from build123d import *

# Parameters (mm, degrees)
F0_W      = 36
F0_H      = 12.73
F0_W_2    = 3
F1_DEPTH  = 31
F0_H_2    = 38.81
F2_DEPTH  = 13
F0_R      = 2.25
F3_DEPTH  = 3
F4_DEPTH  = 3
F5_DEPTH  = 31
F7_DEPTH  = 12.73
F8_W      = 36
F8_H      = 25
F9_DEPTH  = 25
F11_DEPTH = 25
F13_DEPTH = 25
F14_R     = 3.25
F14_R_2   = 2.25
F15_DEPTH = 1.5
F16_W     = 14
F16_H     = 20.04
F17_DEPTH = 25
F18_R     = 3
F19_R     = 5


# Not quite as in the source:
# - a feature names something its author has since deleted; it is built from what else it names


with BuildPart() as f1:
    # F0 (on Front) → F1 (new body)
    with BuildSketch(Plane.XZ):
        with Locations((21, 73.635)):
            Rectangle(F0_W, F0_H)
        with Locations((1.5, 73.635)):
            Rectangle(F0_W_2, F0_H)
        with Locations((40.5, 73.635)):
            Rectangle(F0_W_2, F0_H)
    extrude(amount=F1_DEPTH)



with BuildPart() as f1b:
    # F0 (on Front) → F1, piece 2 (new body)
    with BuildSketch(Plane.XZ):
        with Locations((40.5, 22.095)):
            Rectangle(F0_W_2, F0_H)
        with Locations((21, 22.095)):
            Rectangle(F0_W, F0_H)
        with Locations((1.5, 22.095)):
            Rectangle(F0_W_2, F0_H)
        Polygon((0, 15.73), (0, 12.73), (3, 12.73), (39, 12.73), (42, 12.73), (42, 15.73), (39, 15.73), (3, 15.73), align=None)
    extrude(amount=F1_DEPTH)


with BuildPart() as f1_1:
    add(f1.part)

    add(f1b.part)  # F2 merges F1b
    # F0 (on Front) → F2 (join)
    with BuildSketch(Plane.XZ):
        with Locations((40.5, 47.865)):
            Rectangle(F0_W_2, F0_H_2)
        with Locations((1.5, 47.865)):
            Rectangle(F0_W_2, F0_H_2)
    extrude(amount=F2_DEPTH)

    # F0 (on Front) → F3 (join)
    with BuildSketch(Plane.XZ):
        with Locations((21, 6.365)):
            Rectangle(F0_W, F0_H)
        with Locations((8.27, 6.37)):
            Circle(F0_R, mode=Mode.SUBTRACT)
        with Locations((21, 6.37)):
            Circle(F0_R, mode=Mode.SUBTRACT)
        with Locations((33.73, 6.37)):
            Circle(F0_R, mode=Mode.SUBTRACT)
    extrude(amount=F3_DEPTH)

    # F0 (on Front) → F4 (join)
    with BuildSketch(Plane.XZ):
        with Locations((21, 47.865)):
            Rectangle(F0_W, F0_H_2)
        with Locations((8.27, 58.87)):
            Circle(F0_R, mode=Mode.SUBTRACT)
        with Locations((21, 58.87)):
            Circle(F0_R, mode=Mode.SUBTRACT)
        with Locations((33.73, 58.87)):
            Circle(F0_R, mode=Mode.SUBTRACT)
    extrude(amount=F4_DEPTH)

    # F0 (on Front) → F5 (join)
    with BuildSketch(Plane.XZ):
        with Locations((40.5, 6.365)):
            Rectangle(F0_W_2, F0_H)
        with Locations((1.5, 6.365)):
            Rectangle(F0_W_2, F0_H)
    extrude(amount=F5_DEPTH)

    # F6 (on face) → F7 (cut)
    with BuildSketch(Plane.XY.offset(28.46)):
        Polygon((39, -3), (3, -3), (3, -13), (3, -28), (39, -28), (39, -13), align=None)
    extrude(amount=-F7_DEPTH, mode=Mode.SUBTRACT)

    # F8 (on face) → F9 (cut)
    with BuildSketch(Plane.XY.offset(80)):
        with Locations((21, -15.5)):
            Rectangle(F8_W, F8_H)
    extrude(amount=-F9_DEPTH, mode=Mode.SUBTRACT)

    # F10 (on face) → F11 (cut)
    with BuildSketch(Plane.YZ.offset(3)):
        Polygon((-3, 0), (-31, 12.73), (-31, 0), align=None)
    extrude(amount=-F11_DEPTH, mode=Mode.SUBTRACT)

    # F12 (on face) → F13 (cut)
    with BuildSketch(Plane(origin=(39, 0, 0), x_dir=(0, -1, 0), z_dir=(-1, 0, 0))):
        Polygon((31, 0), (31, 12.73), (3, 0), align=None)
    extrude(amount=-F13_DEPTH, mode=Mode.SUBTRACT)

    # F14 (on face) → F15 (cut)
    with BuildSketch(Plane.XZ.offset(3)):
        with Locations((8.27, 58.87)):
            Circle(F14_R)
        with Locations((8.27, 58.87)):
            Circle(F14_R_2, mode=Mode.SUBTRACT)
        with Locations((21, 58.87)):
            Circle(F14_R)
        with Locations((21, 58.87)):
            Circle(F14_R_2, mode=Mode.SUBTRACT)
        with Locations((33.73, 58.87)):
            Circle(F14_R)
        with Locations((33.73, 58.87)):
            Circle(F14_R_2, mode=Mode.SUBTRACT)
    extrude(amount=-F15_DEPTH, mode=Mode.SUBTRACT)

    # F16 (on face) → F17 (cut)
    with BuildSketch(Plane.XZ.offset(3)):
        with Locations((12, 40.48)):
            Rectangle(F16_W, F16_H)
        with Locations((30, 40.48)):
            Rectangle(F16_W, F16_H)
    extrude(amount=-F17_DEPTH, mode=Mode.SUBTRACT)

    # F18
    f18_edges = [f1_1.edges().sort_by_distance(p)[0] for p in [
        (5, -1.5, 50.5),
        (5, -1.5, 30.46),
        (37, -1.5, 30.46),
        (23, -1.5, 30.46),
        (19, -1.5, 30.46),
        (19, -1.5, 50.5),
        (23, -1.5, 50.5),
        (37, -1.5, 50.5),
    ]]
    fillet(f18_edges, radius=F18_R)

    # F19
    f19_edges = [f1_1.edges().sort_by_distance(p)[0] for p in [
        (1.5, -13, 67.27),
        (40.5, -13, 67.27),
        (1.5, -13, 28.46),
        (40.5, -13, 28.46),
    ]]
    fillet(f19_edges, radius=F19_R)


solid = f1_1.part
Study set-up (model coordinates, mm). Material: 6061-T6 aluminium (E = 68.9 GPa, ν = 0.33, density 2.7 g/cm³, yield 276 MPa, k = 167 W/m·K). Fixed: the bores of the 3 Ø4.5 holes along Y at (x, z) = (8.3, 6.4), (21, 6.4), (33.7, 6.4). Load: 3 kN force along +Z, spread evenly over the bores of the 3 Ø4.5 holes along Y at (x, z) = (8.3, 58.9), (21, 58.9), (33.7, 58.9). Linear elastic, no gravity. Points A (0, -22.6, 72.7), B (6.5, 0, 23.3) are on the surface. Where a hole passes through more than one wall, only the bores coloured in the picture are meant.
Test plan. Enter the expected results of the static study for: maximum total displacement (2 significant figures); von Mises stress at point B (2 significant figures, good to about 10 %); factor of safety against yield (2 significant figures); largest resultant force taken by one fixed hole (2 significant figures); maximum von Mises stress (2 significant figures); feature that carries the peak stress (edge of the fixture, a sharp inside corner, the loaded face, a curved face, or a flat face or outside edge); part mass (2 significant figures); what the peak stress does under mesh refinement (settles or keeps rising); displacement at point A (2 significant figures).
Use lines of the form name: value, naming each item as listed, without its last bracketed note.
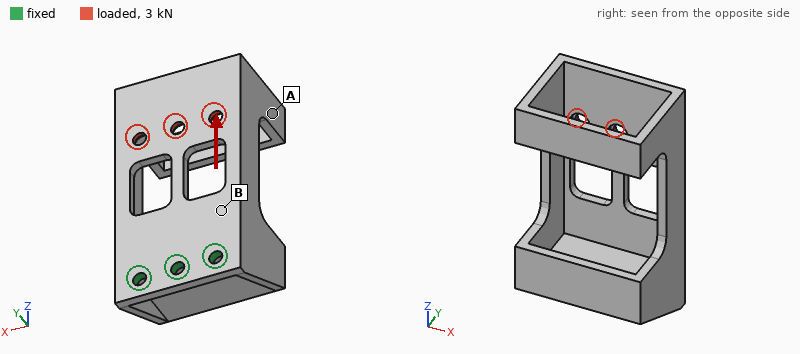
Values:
maximum total displacement: 0.25 mm
von Mises stress at point B: 29 MPa
factor of safety against yield: 1.9
largest resultant force taken by one fixed hole: 1.2 kN
maximum von Mises stress: 150 MPa
feature that carries the peak stress: a curved face
part mass: 60 g
what the peak stress does under mesh refinement: settles
displacement at point A: 0.20 mm
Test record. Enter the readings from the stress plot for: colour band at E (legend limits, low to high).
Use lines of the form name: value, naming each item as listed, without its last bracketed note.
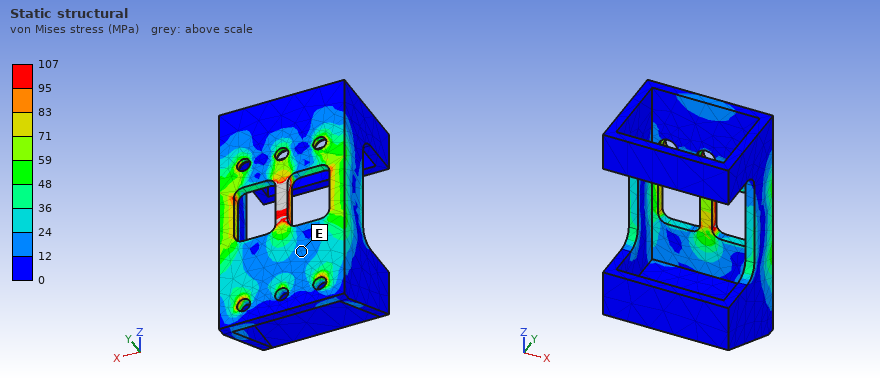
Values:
colour band at E: 12 to 24 MPa
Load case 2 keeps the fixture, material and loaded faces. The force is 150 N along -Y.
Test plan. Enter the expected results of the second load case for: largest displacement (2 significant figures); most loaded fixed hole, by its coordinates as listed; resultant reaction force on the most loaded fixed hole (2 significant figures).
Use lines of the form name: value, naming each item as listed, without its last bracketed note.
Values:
largest displacement: 0.26 mm
most loaded fixed hole, by its coordinates as listed: (21, 6.4)
resultant reaction force on the most loaded fixed hole: 250 N
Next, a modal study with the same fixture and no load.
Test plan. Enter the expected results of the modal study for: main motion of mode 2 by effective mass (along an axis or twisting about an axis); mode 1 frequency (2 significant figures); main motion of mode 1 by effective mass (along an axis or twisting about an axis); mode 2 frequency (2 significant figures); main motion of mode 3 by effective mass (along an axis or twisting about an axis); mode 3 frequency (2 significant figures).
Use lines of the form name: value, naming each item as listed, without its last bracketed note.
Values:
main motion of mode 2 by effective mass: along X
mode 1 frequency: 750 Hz
main motion of mode 1 by effective mass: along Y
mode 2 frequency: 1200 Hz
main motion of mode 3 by effective mass: along X
mode 3 frequency: 2300 Hz
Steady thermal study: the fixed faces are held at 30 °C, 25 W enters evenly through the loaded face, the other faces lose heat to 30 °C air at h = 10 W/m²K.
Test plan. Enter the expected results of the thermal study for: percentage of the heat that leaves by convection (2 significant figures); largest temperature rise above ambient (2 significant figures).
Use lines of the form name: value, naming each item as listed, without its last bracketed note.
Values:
percentage of the heat that leaves by convection: 17 %
largest temperature rise above ambient: 60 K
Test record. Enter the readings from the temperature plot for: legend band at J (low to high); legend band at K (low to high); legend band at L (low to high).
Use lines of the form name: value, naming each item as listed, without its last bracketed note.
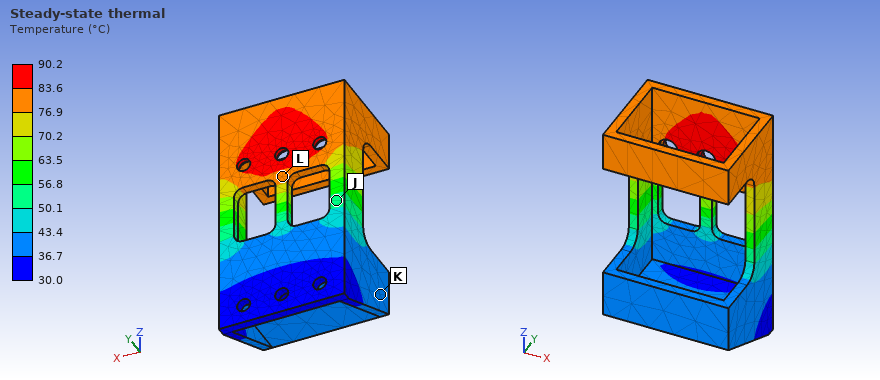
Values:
legend band at J: 50.1 to 56.8 °C
legend band at K: 36.7 to 43.4 °C
legend band at L: 76.9 to 83.6 °C
